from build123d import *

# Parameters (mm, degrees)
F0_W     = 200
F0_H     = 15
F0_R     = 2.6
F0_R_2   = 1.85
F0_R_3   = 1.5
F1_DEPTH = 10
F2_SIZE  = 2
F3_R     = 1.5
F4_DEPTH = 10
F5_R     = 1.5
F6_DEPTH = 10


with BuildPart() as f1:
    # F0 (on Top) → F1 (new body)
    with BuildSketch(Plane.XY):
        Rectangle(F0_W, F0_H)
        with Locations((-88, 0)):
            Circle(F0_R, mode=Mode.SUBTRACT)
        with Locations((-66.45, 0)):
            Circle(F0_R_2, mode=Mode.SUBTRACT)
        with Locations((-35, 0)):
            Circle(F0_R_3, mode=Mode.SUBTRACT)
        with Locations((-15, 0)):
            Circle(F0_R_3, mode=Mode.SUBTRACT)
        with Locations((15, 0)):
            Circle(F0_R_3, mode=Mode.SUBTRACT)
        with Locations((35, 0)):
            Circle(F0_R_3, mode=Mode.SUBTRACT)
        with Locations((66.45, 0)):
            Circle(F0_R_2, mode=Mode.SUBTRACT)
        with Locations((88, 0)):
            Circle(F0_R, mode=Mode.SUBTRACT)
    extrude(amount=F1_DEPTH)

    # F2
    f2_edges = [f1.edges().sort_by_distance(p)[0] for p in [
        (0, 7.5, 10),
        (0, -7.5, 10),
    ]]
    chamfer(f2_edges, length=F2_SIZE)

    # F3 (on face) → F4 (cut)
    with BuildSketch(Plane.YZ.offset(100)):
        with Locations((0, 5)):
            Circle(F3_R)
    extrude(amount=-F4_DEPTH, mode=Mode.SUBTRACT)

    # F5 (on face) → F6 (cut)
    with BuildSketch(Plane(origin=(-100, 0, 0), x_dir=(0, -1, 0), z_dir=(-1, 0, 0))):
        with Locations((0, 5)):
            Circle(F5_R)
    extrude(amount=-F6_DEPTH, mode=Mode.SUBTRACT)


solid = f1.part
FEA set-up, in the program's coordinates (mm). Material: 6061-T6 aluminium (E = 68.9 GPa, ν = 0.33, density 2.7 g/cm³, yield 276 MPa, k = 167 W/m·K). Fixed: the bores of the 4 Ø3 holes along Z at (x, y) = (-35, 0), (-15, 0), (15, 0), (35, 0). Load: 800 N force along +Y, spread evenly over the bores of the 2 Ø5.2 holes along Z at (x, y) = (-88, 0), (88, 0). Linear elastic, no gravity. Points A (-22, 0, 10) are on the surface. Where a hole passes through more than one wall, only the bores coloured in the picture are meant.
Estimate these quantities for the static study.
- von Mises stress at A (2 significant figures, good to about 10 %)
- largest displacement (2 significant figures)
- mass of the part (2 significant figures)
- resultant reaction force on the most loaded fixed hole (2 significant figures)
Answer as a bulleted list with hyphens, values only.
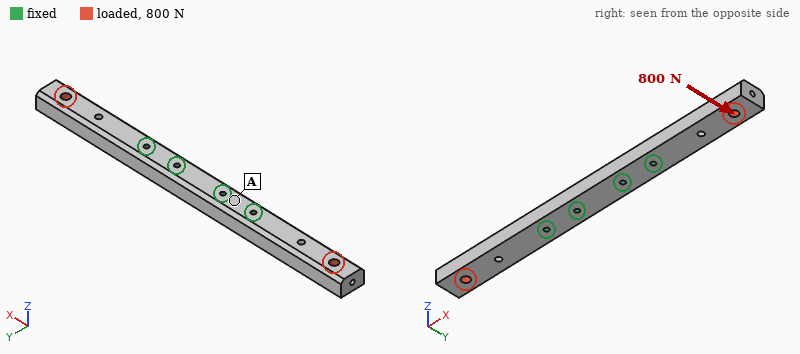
- 13 MPa
- 0.21 mm
- 76 g
- 1.2 kN
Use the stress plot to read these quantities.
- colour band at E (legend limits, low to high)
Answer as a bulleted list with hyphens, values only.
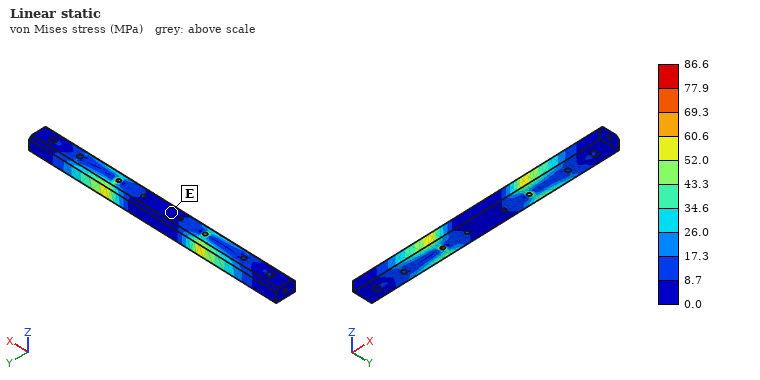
- 0.0 to 8.7 MPa
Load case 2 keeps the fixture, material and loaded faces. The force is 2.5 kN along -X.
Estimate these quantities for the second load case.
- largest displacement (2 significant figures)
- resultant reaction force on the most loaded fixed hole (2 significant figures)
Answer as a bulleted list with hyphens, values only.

- 8.9 µm
- 1.1 kN
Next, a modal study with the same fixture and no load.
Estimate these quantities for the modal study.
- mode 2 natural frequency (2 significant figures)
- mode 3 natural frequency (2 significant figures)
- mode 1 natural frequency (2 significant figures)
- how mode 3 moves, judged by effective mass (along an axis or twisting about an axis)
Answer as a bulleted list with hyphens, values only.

- 1900 Hz
- 2400 Hz
- 1900 Hz
- along Y
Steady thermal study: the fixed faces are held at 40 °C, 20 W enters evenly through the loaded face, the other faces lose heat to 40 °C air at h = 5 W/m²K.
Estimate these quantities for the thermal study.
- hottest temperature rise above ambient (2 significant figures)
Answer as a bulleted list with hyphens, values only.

- 23 K
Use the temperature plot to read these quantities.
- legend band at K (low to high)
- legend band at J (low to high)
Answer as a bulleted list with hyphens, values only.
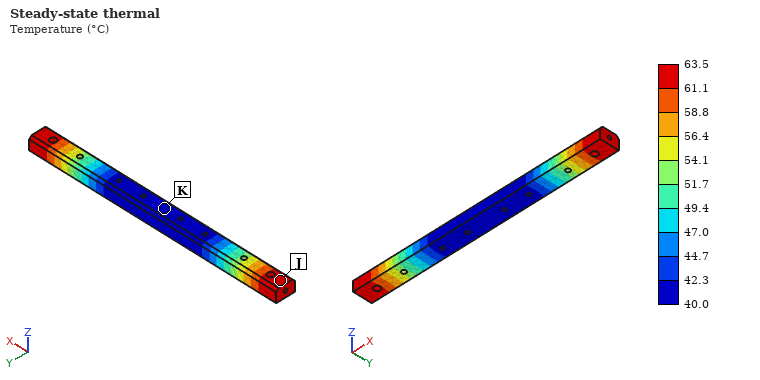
- 40.0 to 42.3 °C
- 61.1 to 63.5 °C
